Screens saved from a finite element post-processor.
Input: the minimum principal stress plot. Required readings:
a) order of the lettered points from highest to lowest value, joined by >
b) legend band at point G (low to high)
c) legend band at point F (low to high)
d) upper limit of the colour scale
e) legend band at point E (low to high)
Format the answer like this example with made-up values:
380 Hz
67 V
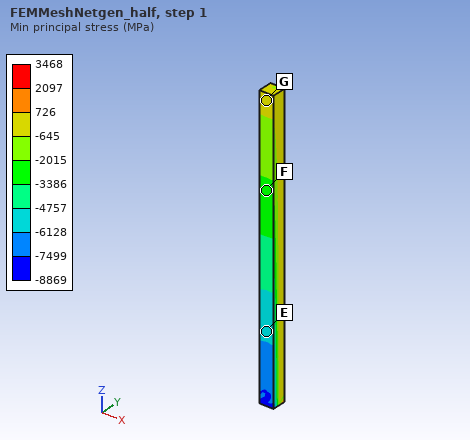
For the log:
G > F > E
-645 to 726 MPa
-3386 to -2015 MPa
3468 MPa
-6128 to -4757 MPa
